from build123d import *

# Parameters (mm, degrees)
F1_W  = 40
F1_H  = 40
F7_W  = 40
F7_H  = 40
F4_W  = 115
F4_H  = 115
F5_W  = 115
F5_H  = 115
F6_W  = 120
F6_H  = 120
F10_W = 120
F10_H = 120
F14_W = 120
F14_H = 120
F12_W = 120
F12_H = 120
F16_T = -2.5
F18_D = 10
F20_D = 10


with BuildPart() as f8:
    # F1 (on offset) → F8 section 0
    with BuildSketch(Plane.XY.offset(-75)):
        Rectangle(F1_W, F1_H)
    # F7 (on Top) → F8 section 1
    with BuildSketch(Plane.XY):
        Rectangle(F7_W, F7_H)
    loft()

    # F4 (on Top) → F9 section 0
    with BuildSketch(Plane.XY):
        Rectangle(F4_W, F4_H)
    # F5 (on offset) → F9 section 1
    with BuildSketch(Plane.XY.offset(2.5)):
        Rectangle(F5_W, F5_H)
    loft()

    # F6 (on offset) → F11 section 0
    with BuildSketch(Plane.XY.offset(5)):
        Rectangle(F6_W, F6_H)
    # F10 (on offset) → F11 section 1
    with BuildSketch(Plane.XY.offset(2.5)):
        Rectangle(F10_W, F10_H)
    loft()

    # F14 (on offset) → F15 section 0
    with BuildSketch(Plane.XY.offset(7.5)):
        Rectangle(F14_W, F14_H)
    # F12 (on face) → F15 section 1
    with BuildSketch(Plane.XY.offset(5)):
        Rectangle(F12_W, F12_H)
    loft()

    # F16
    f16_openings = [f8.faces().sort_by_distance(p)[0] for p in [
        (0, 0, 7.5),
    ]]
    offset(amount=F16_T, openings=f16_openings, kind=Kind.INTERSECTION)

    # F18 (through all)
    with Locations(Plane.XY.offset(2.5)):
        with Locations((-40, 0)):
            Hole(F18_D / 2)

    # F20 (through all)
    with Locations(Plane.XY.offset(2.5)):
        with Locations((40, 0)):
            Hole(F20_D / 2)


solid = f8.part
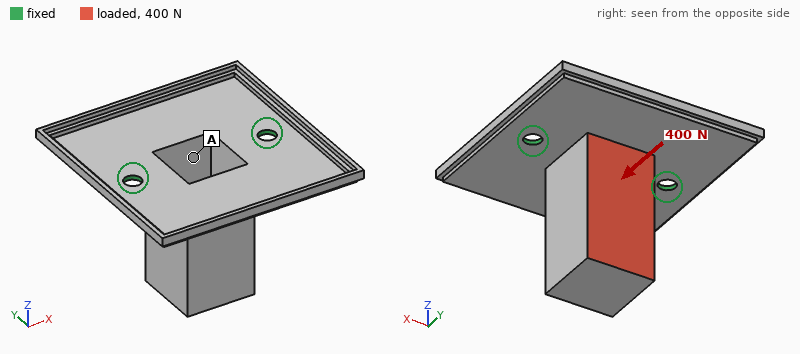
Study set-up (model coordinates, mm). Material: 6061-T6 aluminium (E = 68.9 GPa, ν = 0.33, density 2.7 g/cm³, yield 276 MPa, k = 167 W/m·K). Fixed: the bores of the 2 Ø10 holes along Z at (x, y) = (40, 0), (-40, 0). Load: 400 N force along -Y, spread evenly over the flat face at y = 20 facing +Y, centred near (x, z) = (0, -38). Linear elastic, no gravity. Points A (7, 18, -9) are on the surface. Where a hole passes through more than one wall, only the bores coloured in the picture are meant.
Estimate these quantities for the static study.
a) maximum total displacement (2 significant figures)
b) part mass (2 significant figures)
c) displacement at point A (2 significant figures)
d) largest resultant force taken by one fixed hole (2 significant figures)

0.62 mm
190 g
0.16 mm
200 N
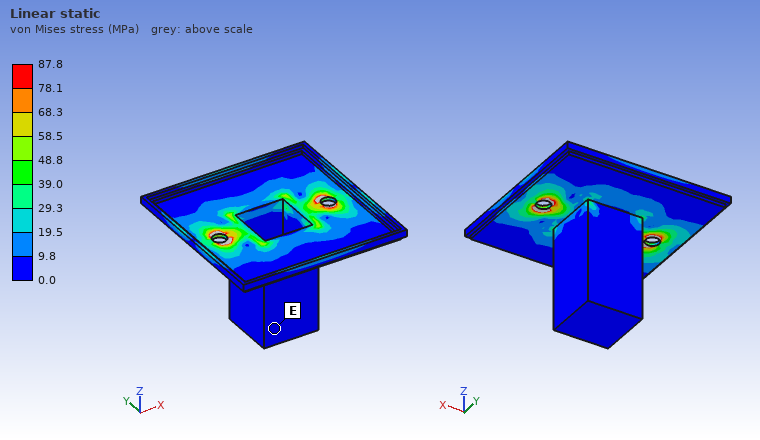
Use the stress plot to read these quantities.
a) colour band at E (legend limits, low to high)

0.0 to 9.8 MPa
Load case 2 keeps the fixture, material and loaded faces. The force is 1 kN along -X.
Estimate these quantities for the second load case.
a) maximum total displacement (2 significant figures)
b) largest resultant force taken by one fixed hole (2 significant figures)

0.34 mm
820 N
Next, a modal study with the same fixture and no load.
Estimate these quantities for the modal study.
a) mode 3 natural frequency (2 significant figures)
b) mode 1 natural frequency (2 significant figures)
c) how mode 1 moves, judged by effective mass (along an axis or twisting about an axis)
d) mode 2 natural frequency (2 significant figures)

980 Hz
400 Hz
along Y
960 Hz
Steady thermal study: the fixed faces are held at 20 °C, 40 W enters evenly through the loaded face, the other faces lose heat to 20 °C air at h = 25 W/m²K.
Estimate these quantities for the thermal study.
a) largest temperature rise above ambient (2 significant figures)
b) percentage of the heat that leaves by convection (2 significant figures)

34 K
45 %
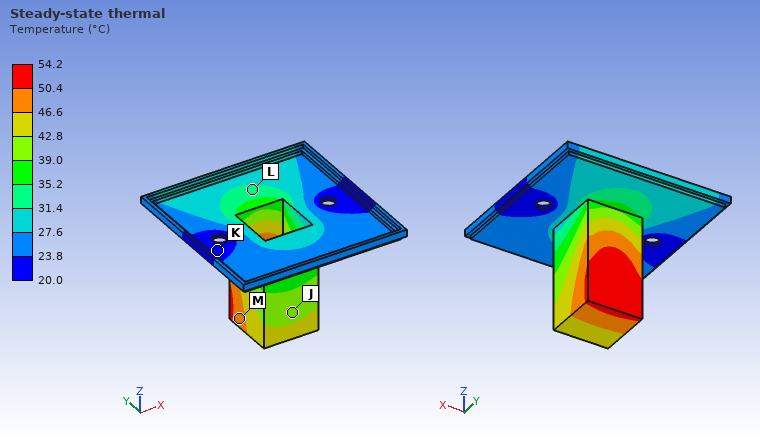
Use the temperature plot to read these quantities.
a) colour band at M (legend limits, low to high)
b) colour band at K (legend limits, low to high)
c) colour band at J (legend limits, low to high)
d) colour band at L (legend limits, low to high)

46.6 to 50.4 °C
20.0 to 23.8 °C
39.0 to 42.8 °C
31.4 to 35.2 °C
